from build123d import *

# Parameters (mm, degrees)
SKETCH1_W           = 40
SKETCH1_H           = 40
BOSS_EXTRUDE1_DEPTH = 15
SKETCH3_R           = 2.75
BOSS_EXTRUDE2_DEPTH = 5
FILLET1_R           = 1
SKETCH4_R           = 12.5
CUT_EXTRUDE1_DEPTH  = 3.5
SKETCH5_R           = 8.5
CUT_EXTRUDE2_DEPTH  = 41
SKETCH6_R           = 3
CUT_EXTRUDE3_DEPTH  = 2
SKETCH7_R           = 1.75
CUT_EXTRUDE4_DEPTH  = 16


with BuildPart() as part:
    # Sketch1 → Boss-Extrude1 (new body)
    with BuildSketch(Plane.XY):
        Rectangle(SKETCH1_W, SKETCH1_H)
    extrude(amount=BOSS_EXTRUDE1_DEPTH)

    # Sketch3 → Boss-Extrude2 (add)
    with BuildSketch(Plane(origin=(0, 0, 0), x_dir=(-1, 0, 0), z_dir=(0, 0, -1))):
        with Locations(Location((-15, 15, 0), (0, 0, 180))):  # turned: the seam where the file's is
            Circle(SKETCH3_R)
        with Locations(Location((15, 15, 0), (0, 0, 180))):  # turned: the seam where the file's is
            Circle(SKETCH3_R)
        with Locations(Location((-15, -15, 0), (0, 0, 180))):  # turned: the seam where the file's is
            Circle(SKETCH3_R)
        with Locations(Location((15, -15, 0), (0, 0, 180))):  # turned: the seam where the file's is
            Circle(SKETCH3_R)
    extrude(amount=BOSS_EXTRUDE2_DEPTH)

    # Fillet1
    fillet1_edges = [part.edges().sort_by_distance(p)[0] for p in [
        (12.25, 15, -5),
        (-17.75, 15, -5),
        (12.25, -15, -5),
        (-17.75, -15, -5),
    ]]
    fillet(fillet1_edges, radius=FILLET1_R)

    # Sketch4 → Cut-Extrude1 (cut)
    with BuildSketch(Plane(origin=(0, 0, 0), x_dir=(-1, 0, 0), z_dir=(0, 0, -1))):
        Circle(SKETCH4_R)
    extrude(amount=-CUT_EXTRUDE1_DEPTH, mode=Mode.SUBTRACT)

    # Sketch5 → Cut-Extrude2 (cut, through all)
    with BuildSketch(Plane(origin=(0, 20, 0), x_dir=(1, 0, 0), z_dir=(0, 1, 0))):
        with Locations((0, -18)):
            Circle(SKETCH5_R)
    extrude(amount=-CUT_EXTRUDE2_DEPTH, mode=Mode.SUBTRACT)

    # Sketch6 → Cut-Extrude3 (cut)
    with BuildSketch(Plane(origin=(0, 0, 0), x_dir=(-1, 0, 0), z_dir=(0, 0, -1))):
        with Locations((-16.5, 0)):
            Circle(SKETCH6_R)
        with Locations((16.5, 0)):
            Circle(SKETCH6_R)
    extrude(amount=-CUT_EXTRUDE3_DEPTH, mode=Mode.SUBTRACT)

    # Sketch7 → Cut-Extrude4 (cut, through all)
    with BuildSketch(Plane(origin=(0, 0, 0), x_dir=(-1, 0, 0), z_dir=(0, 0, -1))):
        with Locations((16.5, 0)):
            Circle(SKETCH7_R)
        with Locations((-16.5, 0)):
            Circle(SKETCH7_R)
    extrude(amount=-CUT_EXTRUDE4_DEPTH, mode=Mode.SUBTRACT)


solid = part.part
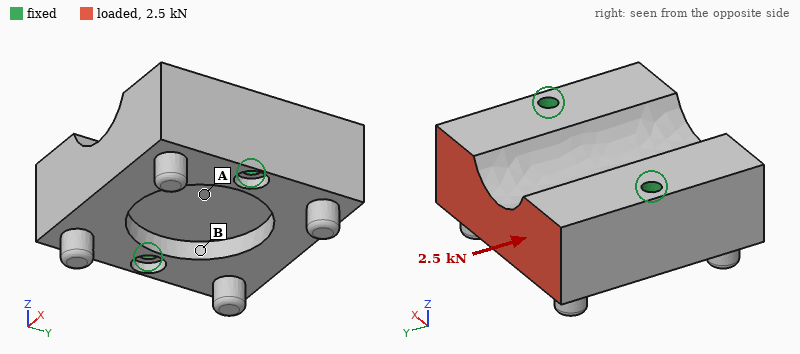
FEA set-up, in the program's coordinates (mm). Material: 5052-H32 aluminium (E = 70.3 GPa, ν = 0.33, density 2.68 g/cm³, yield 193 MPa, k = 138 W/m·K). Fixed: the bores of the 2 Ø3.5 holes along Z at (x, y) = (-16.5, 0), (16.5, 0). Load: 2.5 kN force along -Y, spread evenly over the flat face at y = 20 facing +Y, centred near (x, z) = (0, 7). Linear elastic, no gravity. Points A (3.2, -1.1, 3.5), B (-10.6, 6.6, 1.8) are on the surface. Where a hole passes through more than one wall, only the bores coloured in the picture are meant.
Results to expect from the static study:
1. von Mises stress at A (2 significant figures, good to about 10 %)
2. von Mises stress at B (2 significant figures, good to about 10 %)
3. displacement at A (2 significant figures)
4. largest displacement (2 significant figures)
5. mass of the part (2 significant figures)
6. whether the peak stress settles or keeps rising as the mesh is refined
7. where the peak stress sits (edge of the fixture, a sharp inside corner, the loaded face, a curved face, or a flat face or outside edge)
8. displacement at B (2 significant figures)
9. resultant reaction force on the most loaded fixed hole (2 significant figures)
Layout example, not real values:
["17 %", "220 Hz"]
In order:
["3.6 MPa", "9.5 MPa", "1.4 µm", "4.3 µm", "53 g", "keeps rising", "edge of the fixture", "1.8 µm", "1.3 kN"]
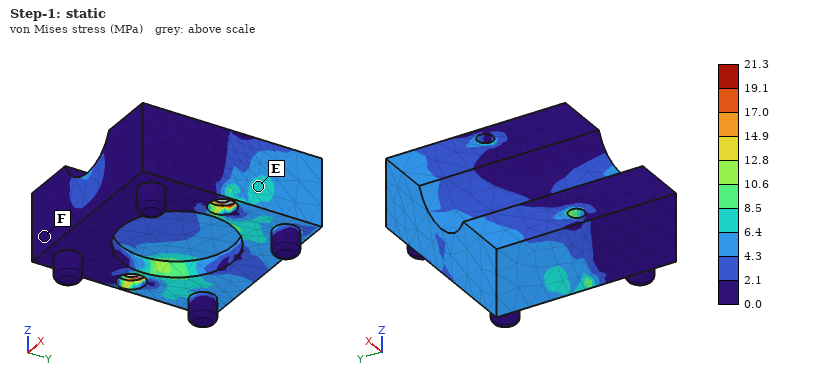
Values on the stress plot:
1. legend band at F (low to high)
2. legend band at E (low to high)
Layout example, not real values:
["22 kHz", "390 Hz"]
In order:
["0.0 to 2.1 MPa", "6.4 to 8.5 MPa"]
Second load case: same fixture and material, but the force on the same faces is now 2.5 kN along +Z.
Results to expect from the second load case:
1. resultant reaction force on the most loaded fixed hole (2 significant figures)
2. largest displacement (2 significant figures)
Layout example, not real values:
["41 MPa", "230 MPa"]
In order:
["1.3 kN", "32 µm"]
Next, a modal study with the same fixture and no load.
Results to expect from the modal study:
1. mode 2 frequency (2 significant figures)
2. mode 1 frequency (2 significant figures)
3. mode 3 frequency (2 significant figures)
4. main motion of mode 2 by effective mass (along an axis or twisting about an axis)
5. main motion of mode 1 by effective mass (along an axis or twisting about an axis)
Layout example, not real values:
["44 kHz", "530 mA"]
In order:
["17 kHz", "14 kHz", "21 kHz", "along Z", "twisting about X"]
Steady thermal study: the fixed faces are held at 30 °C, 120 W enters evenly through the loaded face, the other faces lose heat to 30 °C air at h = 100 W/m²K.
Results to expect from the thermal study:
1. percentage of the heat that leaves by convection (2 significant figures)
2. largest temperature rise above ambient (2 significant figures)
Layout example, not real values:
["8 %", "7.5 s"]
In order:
["6.0 %", "41 K"]
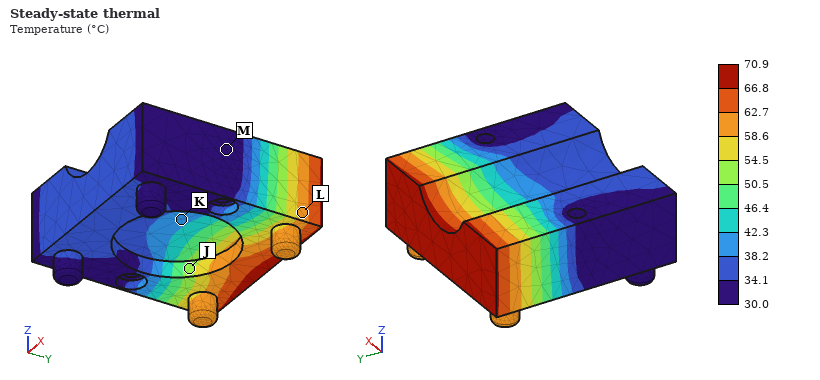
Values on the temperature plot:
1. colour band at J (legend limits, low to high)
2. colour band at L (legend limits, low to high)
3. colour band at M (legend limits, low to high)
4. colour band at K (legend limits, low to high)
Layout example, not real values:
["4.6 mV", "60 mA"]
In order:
["50.5 to 54.5 °C", "58.6 to 62.7 °C", "30.0 to 34.1 °C", "38.2 to 42.3 °C"]
